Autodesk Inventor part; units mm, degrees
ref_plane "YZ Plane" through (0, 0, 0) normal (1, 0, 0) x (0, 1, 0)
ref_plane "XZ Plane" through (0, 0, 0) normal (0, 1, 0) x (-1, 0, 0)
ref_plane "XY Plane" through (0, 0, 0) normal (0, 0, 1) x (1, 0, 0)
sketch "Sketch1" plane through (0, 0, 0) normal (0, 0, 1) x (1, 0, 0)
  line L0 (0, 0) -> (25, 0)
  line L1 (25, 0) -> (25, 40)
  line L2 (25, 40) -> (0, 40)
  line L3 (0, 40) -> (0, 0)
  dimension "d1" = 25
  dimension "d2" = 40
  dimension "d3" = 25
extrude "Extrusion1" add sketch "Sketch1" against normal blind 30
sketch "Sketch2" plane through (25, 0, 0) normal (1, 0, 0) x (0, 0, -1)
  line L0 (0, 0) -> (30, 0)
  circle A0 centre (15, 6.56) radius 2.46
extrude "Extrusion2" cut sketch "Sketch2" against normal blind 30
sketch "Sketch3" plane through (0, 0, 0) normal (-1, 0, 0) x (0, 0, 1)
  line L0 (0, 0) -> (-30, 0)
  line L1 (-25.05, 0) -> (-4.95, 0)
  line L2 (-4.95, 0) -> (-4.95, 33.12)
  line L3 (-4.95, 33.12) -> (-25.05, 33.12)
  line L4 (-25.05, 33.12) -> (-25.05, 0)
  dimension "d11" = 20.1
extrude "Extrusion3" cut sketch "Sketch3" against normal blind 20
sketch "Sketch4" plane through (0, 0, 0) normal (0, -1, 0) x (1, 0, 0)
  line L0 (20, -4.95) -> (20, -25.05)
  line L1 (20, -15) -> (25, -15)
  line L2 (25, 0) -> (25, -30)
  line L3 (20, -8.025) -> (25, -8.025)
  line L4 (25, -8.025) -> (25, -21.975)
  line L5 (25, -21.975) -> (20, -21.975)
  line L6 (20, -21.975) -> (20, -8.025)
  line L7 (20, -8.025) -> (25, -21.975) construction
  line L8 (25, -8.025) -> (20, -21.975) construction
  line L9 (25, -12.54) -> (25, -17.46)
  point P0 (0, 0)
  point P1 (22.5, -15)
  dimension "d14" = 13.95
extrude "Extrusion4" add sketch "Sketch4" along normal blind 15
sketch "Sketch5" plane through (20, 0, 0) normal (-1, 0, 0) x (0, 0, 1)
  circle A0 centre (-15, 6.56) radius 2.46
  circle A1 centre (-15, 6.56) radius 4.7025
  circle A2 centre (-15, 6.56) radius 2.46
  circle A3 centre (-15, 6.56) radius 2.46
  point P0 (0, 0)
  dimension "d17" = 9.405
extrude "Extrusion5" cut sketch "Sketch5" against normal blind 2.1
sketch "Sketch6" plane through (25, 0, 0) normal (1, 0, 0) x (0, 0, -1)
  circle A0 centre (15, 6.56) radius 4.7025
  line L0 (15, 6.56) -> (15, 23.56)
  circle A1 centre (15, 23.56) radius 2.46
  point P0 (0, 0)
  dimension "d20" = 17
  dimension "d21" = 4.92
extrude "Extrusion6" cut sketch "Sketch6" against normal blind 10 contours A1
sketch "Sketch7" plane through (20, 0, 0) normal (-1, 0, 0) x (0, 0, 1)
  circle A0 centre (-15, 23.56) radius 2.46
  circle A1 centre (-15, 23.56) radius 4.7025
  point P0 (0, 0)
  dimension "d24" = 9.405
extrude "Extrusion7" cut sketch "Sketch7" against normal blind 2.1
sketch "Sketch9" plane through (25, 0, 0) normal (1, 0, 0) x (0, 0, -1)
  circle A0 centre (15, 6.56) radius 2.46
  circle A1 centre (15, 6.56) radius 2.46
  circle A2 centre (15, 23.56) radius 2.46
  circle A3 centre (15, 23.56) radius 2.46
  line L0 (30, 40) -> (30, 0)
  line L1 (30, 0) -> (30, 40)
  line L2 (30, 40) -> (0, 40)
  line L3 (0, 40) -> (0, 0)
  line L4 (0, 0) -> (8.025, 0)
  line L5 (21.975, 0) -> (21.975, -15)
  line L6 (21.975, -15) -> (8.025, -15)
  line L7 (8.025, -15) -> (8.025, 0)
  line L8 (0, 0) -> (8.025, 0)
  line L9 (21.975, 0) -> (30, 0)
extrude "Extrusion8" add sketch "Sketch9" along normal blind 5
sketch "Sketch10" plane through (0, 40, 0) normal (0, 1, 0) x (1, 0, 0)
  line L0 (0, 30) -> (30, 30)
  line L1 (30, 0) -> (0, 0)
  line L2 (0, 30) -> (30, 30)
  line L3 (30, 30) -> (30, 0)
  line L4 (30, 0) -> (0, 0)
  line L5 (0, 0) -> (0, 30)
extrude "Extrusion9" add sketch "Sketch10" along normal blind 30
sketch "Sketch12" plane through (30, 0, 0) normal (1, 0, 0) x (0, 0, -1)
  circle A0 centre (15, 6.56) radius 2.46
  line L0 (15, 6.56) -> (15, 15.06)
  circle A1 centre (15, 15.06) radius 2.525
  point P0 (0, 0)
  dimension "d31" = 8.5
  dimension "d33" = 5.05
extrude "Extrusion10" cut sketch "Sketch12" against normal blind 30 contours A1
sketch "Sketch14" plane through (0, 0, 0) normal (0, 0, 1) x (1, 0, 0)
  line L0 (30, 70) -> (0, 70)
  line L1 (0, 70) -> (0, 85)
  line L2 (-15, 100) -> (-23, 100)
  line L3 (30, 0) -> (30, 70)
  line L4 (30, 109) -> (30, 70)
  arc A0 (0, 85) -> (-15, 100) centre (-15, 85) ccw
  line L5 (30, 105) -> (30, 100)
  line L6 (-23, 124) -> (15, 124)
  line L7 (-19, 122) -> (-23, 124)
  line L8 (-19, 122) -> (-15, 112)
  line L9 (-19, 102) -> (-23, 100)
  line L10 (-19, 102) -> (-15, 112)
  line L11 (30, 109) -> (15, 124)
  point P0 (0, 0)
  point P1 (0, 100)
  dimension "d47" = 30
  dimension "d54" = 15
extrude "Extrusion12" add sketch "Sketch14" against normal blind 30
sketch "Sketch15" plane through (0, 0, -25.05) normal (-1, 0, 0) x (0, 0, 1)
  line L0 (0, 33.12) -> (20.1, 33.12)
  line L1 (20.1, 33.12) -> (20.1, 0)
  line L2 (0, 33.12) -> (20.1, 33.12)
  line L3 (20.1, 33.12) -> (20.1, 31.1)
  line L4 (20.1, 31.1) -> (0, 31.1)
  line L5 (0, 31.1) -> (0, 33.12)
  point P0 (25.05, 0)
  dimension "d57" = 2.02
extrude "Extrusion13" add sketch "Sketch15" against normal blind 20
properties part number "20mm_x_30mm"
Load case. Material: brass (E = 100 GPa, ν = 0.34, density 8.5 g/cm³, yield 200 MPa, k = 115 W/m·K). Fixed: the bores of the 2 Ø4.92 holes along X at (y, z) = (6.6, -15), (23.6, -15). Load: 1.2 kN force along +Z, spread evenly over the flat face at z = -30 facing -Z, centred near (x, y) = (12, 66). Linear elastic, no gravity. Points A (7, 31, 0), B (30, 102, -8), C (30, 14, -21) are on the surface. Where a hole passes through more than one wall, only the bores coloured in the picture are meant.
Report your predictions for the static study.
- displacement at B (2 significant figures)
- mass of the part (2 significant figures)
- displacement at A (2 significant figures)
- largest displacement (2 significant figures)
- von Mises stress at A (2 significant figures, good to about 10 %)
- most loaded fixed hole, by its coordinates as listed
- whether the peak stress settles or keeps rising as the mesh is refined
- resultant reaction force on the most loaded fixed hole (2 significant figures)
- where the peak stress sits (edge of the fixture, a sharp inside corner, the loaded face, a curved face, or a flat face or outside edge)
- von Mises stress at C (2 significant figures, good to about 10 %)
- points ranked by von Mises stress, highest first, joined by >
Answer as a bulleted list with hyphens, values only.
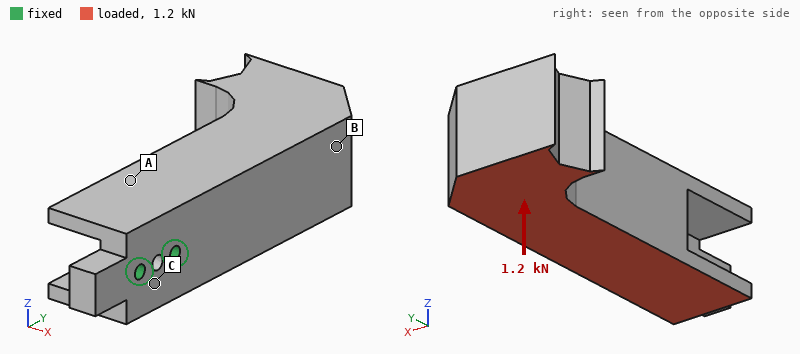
- 51 µm
- 950 g
- 14 µm
- 89 µm
- 12 MPa
- (23.6, -15)
- keeps rising
- 3.3 kN
- edge of the fixture
- 24 MPa
- C > A > B
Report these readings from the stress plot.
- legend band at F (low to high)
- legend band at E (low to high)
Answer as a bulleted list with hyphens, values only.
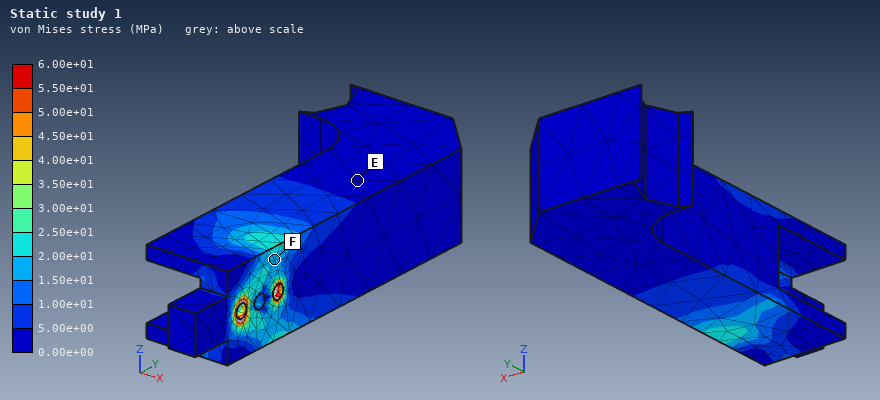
- 1.50e+01 to 2.00e+01 MPa
- 0.00e+00 to 5.00e+00 MPa
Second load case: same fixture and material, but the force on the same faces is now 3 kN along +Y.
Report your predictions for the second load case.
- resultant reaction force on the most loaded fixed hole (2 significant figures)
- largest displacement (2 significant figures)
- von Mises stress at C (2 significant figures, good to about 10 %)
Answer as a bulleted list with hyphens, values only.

- 3.1 kN
- 97 µm
- 9.8 MPa
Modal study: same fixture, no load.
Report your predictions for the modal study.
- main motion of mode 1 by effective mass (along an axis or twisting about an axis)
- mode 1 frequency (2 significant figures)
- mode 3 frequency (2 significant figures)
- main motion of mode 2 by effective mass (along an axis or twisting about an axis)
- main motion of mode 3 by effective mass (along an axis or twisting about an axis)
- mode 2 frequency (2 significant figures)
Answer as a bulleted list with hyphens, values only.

- along X
- 620 Hz
- 1900 Hz
- along Z
- twisting about Y
- 730 Hz
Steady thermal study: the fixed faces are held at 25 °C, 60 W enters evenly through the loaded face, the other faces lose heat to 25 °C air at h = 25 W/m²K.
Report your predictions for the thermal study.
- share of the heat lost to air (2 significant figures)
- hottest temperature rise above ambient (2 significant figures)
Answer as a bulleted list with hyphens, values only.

- 15 %
- 35 K
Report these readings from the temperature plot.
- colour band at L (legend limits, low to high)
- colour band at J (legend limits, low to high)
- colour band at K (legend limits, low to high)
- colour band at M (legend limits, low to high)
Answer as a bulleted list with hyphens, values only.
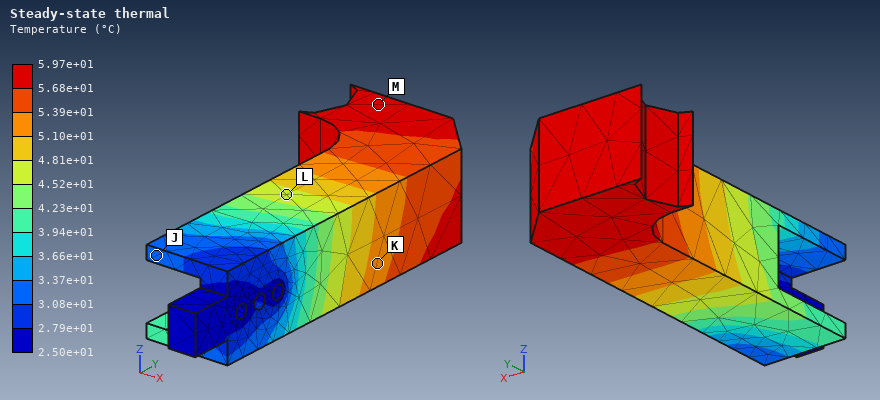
- 4.52e+01 to 4.81e+01 °C
- 3.08e+01 to 3.37e+01 °C
- 5.10e+01 to 5.39e+01 °C
- 5.68e+01 to 5.97e+01 °C
